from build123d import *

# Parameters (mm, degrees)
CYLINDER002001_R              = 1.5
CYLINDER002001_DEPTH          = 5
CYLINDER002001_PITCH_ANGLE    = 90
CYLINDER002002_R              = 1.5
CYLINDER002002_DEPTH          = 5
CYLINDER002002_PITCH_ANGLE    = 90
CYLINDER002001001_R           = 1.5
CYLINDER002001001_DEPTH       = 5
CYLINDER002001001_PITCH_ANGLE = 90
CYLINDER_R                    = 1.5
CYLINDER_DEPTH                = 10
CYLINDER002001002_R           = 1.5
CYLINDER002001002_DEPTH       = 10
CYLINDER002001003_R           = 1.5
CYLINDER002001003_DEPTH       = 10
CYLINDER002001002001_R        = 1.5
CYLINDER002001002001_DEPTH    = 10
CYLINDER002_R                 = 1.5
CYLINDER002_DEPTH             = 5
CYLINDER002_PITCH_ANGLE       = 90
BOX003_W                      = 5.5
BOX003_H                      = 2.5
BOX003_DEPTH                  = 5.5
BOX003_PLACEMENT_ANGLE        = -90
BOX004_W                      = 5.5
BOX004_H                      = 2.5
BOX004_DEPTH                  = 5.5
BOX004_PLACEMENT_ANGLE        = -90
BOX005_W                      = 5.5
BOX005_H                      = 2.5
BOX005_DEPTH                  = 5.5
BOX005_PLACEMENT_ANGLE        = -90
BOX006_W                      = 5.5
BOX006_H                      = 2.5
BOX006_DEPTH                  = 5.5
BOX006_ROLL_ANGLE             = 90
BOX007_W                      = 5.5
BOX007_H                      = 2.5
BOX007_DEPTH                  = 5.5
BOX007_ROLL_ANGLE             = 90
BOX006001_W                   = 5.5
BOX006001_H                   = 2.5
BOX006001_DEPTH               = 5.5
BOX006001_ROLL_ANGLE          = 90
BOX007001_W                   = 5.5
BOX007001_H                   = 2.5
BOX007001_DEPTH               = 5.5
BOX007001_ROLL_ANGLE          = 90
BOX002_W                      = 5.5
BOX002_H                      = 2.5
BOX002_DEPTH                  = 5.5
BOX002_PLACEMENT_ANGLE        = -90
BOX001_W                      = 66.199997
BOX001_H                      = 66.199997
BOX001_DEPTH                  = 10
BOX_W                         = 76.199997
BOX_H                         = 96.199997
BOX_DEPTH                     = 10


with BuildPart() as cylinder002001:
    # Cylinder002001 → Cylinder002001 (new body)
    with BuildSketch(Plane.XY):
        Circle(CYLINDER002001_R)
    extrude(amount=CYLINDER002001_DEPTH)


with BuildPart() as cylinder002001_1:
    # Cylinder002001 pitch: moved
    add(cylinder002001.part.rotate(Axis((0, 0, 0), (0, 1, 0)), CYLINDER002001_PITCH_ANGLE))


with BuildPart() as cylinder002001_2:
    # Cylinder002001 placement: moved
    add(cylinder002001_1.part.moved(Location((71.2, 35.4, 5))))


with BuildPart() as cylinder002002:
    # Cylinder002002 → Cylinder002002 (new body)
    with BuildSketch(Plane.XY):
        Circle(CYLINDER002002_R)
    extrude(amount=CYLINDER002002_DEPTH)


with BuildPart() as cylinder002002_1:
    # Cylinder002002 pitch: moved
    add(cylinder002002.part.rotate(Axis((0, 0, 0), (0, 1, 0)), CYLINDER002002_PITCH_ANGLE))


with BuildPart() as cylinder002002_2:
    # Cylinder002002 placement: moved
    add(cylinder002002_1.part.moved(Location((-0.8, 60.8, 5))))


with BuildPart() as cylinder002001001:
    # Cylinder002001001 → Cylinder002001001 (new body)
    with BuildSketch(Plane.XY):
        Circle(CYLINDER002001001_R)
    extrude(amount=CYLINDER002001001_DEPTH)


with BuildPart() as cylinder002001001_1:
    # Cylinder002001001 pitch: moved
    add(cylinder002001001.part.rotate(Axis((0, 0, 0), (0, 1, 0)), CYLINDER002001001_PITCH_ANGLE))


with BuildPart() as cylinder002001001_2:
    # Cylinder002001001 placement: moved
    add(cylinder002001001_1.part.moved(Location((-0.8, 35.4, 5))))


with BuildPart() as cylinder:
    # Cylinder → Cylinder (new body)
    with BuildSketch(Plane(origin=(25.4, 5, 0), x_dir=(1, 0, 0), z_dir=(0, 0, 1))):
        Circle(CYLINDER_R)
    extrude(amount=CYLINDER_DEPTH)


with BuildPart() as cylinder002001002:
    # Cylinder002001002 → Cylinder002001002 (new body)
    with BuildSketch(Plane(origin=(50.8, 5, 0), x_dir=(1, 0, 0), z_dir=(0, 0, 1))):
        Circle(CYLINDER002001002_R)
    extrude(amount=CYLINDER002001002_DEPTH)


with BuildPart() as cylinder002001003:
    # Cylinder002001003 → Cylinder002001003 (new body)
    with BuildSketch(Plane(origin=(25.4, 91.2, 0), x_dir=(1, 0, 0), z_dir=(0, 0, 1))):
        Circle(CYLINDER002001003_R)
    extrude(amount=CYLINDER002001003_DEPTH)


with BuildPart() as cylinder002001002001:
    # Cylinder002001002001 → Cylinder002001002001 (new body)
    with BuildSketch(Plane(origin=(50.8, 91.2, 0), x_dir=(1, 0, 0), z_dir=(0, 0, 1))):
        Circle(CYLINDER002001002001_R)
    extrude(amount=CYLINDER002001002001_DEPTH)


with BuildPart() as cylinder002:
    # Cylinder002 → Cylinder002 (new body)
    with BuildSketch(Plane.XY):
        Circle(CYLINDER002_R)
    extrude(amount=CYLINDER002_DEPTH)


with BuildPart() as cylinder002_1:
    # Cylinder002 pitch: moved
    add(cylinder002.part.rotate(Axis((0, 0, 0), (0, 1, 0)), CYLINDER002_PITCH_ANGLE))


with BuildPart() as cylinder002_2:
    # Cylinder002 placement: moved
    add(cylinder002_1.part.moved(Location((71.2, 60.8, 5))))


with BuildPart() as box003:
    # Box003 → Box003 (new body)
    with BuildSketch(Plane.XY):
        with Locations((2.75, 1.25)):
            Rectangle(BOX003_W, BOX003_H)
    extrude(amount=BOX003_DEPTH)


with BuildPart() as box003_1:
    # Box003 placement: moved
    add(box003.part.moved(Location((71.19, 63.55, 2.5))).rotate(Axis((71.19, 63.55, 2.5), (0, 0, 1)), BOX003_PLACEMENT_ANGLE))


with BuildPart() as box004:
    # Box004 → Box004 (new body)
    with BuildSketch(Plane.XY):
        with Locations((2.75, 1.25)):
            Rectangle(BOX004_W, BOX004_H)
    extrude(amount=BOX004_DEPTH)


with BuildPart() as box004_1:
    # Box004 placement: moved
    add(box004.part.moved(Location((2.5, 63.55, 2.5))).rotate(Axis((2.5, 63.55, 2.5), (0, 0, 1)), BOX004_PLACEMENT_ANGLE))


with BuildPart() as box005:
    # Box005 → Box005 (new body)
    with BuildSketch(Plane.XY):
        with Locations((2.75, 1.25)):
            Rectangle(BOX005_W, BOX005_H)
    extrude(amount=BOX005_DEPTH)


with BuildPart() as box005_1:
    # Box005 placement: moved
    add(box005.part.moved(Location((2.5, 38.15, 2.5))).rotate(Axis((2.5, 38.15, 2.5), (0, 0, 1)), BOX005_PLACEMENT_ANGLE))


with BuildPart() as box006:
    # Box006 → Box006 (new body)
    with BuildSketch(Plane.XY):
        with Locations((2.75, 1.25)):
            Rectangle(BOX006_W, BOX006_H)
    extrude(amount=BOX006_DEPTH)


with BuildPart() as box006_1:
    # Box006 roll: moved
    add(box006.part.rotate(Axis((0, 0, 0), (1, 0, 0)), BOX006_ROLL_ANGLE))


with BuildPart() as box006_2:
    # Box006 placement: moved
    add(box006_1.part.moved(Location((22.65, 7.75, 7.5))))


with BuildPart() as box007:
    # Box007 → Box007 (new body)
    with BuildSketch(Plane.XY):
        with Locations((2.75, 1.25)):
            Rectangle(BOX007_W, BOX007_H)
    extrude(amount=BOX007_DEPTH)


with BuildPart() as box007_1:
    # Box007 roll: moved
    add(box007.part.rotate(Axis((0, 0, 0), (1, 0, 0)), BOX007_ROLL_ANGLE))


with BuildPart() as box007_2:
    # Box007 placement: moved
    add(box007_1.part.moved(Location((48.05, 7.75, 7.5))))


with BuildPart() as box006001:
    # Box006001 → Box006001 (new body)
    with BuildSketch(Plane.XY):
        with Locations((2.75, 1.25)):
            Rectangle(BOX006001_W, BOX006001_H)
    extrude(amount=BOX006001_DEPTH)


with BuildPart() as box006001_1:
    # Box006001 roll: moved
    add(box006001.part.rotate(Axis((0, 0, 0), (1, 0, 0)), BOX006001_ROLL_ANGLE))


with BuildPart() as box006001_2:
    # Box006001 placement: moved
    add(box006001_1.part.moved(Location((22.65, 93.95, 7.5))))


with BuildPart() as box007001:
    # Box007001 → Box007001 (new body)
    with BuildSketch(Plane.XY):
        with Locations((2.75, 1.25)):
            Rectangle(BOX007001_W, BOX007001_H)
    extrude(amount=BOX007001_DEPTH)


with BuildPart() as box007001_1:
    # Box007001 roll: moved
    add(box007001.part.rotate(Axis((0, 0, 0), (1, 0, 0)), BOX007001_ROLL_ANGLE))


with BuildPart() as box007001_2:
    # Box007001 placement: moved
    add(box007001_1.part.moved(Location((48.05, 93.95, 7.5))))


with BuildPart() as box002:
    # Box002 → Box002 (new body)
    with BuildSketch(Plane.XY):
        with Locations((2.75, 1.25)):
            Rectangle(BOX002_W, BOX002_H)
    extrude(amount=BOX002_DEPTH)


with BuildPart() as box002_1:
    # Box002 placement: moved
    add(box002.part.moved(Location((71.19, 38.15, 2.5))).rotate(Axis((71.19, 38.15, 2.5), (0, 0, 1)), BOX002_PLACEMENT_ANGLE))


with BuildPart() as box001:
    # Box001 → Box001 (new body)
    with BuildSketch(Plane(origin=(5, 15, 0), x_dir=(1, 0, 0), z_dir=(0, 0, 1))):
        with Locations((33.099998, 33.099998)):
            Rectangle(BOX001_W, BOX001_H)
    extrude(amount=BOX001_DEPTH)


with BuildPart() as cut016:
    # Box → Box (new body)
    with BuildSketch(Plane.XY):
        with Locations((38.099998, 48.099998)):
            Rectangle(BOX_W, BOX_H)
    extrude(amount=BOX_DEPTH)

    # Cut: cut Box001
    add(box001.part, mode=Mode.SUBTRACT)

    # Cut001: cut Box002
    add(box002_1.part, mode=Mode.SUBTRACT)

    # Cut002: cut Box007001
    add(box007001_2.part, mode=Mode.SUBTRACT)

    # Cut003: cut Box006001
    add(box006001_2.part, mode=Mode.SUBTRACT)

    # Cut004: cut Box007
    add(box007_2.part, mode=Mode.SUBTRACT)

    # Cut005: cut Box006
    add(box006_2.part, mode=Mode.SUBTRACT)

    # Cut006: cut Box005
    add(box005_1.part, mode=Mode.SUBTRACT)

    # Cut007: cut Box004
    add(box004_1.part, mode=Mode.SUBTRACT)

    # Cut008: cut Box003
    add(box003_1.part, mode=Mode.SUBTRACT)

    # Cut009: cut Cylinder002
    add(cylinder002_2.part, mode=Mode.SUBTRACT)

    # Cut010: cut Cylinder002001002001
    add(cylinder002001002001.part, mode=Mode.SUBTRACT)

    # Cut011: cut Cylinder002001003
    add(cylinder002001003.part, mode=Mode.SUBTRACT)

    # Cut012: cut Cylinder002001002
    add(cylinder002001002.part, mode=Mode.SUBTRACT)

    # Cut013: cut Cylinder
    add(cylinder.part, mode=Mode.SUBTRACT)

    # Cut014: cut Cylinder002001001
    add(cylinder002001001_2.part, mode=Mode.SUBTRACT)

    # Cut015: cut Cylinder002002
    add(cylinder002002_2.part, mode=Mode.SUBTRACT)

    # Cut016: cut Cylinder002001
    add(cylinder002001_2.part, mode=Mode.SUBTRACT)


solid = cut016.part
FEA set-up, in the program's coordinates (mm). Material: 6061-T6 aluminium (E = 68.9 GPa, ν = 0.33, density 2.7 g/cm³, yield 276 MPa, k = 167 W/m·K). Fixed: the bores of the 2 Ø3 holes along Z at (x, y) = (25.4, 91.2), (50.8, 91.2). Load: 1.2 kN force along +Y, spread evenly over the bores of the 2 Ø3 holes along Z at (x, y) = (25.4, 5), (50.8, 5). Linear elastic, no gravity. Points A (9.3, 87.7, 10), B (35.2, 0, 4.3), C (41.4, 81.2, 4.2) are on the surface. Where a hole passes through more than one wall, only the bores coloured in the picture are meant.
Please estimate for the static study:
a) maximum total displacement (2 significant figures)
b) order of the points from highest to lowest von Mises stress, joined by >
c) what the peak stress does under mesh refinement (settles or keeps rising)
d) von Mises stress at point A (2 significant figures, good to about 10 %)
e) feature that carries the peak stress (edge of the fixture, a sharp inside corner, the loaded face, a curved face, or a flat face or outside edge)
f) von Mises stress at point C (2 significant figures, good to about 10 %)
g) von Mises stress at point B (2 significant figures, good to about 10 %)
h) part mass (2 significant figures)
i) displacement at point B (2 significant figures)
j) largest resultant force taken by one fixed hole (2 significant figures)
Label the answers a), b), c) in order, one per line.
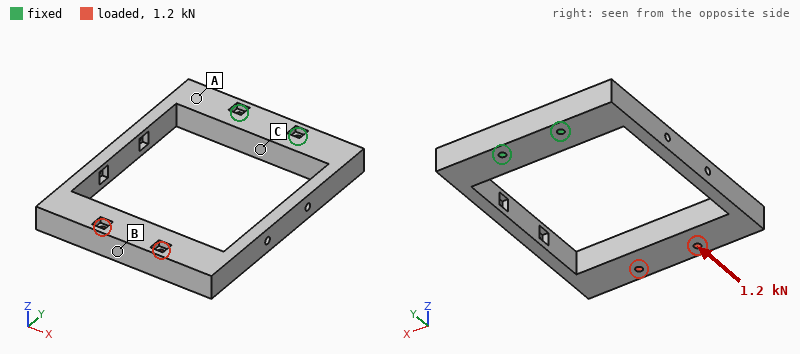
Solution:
a) 0.15 mm
b) B > C > A
c) keeps rising
d) 7.4 MPa
e) edge of the fixture
f) 27 MPa
g) 36 MPa
h) 77 g
i) 0.14 mm
j) 1.0 kN
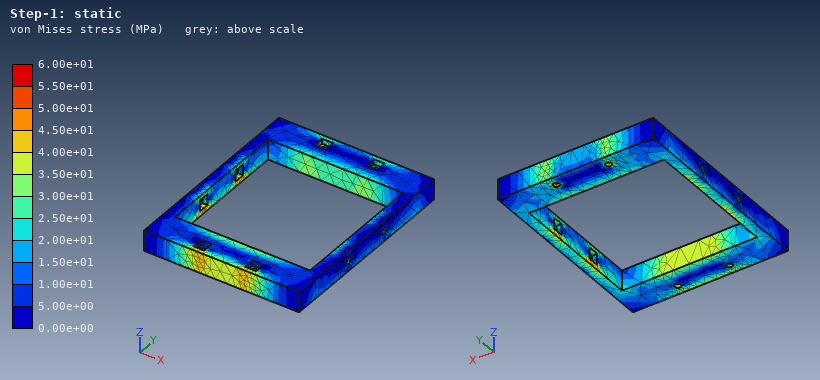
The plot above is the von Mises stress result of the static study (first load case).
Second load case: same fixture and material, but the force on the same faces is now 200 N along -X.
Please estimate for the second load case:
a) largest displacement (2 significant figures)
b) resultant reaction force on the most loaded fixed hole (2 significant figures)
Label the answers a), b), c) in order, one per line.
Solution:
a) 0.52 mm
b) 570 N
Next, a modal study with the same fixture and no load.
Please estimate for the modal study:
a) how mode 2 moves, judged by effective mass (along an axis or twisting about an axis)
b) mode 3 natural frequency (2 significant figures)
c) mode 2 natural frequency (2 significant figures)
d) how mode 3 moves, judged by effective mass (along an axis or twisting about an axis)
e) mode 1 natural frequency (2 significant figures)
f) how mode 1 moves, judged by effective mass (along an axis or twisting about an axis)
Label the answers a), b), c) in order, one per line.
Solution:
a) along X
b) 1100 Hz
c) 520 Hz
d) twisting about Y
e) 430 Hz
f) along Z
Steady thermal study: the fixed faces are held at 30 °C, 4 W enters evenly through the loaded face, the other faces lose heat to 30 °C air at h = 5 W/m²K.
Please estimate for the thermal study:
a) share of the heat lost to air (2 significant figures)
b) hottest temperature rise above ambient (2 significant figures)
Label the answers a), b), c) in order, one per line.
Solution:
a) 16 %
b) 21 K
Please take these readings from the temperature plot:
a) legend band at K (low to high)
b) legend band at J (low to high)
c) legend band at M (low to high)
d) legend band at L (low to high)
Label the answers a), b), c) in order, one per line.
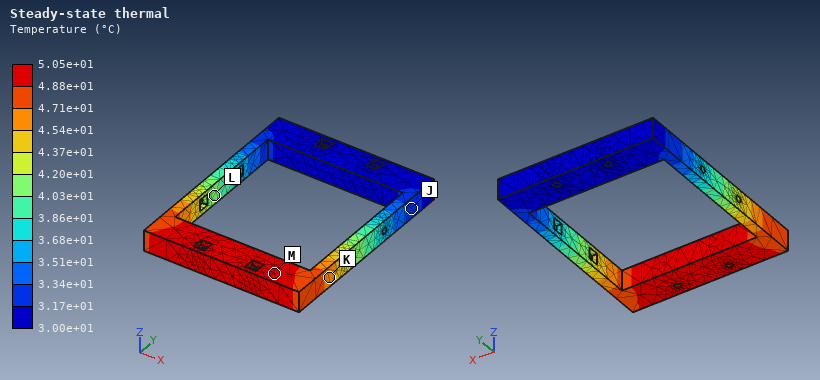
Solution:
a) 4.54e+01 to 4.71e+01 °C
b) 3.17e+01 to 3.34e+01 °C
c) 4.88e+01 to 5.05e+01 °C
d) 4.03e+01 to 4.20e+01 °C
